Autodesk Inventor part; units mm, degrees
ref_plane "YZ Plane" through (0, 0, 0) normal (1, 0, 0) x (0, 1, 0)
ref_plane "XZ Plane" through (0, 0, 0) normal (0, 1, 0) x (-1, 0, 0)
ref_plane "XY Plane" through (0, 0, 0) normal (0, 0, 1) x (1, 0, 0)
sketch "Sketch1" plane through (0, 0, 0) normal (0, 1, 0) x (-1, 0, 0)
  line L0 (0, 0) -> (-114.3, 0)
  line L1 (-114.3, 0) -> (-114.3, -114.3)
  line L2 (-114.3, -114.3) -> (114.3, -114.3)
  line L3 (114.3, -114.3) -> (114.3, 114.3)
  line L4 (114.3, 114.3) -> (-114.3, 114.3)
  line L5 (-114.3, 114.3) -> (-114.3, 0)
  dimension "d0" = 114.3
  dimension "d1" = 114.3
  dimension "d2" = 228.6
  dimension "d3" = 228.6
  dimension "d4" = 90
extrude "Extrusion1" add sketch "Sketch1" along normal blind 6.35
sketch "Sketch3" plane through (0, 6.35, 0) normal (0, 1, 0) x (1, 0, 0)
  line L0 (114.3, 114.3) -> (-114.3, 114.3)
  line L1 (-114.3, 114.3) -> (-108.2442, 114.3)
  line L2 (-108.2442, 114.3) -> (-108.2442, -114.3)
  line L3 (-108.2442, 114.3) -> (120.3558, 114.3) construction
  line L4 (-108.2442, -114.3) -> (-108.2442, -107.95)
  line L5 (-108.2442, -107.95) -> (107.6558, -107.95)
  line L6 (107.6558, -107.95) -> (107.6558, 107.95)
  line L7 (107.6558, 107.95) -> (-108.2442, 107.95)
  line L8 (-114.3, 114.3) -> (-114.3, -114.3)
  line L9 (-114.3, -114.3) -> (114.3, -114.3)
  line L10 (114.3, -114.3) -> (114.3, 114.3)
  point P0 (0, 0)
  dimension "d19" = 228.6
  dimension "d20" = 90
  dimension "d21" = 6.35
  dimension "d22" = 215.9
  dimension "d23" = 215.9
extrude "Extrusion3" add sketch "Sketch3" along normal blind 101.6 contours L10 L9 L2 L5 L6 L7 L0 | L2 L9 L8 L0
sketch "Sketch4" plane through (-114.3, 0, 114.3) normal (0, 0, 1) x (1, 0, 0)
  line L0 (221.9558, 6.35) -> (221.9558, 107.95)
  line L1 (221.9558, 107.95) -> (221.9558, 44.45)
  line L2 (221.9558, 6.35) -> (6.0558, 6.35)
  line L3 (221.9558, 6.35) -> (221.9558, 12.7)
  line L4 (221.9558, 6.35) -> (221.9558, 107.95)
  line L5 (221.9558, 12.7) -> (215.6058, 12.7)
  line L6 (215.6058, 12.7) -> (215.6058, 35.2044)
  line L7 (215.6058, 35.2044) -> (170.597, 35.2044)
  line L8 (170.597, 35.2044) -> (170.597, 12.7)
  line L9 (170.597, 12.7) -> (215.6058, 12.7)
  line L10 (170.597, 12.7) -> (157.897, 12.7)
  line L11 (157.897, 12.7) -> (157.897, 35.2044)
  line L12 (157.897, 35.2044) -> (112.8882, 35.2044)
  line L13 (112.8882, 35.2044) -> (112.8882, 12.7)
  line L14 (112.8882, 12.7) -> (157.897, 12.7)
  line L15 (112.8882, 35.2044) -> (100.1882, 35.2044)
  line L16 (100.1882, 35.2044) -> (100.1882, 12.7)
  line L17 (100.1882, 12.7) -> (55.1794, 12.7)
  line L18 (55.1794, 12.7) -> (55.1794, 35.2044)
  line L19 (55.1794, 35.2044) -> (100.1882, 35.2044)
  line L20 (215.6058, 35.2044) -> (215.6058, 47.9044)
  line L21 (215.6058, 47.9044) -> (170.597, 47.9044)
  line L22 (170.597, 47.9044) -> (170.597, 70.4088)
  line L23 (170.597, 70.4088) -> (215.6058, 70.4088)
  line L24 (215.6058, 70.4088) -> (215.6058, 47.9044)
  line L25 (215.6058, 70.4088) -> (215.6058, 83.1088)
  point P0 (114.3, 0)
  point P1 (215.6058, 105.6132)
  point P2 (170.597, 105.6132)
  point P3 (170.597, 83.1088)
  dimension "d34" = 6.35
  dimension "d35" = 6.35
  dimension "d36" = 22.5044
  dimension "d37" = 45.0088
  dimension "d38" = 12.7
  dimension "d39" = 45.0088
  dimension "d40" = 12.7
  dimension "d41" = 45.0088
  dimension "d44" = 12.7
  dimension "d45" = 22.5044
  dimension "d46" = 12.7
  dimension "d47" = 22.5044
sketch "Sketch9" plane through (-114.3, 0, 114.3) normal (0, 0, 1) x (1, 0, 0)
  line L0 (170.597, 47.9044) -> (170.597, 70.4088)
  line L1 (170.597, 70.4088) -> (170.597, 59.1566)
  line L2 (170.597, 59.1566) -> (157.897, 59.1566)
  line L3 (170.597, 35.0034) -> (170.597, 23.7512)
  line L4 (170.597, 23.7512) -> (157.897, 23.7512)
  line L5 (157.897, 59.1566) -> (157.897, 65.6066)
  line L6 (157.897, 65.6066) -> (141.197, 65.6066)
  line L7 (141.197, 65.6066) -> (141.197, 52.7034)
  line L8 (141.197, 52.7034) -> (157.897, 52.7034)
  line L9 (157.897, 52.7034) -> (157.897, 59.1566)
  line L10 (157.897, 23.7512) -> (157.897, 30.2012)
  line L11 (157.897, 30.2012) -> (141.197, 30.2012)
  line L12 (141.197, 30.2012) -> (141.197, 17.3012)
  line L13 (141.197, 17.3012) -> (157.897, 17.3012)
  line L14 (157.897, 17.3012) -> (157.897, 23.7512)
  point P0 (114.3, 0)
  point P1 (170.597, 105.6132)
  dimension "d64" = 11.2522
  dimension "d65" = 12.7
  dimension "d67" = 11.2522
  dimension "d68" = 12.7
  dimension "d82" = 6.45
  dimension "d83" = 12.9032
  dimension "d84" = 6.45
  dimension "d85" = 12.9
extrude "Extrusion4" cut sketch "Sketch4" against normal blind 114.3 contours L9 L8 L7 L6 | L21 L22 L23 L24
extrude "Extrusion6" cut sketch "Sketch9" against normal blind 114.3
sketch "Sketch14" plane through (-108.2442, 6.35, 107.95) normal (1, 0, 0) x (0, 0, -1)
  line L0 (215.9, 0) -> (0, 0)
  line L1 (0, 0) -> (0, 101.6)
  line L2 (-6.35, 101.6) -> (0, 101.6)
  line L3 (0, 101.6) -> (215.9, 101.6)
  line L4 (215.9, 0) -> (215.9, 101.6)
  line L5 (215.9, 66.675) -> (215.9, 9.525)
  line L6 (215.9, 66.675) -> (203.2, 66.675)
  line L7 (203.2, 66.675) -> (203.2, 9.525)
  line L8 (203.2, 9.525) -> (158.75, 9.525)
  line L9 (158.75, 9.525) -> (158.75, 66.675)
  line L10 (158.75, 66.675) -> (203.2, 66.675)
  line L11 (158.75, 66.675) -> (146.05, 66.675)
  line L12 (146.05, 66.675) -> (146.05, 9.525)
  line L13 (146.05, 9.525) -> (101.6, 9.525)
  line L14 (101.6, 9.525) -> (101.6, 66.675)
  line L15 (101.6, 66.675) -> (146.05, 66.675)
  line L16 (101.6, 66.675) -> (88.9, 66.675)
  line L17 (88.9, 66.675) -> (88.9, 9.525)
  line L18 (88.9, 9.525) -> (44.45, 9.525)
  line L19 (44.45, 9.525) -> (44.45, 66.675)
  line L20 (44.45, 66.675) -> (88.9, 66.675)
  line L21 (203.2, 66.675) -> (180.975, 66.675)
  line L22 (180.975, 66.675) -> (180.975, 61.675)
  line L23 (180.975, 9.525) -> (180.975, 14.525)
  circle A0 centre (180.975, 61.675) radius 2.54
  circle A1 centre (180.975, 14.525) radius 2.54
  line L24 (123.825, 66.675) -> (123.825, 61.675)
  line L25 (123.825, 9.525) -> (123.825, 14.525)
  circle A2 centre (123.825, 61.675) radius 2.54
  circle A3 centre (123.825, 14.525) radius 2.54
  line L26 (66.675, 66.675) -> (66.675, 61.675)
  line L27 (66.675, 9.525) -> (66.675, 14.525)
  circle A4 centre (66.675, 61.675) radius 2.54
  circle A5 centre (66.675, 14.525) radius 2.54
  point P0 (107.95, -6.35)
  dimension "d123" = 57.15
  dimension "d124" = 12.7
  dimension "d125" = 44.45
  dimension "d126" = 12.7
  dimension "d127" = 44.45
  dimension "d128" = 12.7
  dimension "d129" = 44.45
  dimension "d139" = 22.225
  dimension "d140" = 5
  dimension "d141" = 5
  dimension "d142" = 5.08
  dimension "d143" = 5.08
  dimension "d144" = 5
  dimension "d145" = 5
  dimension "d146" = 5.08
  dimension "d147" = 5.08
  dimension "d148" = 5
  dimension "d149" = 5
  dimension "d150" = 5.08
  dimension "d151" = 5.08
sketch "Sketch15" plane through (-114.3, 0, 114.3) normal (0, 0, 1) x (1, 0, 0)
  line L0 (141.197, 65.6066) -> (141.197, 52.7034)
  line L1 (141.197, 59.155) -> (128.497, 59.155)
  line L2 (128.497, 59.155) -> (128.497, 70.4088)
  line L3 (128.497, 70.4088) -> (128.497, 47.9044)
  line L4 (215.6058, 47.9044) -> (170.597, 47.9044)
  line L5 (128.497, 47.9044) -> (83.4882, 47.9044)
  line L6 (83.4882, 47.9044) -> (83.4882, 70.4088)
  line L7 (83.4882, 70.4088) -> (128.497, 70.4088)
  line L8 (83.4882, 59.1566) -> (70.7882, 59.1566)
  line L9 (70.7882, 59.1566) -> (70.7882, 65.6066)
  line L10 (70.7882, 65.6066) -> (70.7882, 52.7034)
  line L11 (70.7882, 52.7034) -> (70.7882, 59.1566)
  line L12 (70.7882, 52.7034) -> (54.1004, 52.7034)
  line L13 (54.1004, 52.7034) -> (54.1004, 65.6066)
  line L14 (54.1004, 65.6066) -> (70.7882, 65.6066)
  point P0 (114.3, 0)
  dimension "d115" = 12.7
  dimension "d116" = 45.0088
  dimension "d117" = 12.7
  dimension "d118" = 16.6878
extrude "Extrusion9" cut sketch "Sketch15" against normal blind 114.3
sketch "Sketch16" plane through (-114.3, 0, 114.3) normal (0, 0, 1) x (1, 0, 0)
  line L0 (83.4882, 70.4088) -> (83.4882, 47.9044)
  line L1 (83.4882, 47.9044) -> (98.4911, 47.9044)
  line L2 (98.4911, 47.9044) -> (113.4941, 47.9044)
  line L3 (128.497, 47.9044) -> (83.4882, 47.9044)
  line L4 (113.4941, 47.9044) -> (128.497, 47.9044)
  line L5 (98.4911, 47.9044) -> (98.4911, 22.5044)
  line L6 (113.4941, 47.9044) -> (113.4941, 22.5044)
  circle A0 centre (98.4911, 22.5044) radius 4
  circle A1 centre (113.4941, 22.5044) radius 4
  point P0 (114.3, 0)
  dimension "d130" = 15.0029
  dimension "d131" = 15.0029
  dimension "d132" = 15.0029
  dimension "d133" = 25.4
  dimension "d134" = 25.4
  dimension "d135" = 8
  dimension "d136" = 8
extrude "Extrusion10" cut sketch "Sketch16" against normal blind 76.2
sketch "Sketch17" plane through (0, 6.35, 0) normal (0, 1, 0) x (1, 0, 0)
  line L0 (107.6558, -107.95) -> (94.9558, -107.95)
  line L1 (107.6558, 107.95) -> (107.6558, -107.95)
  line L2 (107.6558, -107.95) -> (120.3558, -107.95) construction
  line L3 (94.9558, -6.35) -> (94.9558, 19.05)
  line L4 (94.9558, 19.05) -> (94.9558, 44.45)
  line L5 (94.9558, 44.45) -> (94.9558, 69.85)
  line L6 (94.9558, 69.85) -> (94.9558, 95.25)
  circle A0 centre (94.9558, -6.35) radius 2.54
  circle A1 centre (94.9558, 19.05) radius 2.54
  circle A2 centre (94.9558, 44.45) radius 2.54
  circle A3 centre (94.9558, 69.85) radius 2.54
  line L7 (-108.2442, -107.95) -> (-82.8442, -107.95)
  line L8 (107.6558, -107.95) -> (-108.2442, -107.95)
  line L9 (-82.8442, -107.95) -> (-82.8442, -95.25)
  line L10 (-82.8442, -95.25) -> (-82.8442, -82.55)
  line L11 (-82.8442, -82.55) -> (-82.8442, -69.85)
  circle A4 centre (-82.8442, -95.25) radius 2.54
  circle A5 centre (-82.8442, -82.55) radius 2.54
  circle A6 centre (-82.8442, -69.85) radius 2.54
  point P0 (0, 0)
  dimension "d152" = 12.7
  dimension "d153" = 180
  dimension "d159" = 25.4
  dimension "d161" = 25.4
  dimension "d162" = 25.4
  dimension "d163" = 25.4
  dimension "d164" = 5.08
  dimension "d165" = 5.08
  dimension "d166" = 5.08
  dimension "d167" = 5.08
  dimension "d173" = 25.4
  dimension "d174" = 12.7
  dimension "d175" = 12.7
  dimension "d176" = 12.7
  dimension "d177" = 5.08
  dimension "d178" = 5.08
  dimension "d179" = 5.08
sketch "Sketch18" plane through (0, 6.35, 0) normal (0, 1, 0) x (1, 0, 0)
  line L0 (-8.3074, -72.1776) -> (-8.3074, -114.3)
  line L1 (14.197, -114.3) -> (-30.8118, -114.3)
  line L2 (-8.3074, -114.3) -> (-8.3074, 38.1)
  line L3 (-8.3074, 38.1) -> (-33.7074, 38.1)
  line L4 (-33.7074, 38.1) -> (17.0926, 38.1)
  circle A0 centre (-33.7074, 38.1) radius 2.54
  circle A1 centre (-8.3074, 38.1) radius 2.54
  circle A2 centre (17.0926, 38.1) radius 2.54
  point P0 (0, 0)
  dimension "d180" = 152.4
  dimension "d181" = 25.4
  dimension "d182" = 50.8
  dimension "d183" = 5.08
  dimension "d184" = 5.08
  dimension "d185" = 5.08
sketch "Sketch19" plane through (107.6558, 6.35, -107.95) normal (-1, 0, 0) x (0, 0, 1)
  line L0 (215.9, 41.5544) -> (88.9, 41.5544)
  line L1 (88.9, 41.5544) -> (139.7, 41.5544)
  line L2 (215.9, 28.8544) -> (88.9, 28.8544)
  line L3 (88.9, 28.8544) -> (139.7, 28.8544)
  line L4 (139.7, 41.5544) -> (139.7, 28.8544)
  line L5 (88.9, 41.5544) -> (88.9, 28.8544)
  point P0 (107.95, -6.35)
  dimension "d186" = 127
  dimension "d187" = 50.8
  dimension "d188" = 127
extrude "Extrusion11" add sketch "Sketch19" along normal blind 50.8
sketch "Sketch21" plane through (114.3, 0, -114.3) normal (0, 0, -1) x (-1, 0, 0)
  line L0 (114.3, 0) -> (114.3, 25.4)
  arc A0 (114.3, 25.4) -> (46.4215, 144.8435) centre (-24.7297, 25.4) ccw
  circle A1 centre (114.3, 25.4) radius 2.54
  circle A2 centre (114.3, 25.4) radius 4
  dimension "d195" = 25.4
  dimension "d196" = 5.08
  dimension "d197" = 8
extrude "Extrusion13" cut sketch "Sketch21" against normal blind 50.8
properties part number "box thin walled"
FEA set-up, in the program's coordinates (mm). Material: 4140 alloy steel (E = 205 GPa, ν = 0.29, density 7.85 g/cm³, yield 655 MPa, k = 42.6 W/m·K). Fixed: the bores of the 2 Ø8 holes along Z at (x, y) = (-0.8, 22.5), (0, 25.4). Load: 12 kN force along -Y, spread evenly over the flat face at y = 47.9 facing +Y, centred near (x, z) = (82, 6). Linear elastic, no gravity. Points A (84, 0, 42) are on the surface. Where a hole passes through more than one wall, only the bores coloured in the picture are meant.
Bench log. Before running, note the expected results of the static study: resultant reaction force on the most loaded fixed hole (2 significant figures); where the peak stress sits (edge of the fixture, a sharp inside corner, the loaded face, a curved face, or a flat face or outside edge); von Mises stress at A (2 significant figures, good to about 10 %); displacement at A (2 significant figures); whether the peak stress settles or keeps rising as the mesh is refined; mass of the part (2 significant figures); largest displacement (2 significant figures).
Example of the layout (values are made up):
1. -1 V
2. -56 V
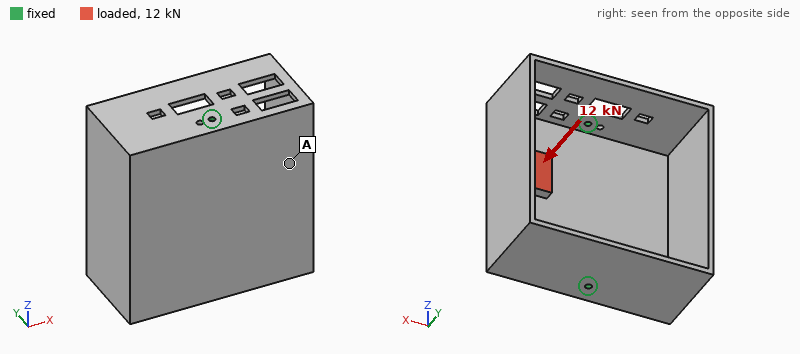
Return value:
1. 6.3 kN
2. edge of the fixture
3. 41 MPa
4. 0.55 mm
5. keeps rising
6. 7.2 kg
7. 1.1 mm
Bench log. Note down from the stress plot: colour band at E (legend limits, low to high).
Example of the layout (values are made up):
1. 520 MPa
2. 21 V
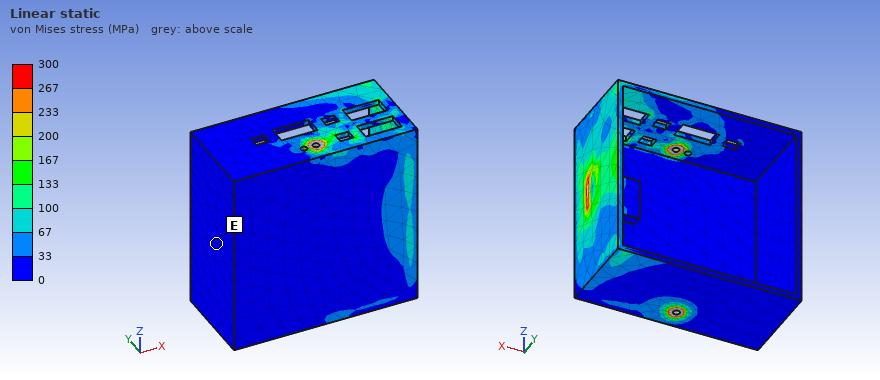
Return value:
1. 0 to 33 MPa
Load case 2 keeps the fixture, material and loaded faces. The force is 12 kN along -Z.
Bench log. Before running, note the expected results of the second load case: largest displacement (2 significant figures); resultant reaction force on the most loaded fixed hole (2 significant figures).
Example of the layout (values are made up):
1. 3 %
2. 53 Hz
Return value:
1. 0.58 mm
2. 7.9 kN
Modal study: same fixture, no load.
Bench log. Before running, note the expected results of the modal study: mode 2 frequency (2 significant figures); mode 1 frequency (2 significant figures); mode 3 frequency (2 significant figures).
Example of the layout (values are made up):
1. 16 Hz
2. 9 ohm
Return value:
1. 400 Hz
2. 290 Hz
3. 670 Hz
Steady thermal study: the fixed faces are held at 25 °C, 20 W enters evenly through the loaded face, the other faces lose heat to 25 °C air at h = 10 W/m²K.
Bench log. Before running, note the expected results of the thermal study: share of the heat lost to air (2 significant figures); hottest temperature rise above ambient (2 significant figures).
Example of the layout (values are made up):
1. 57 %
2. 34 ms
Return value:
1. 83 %
2. 45 K
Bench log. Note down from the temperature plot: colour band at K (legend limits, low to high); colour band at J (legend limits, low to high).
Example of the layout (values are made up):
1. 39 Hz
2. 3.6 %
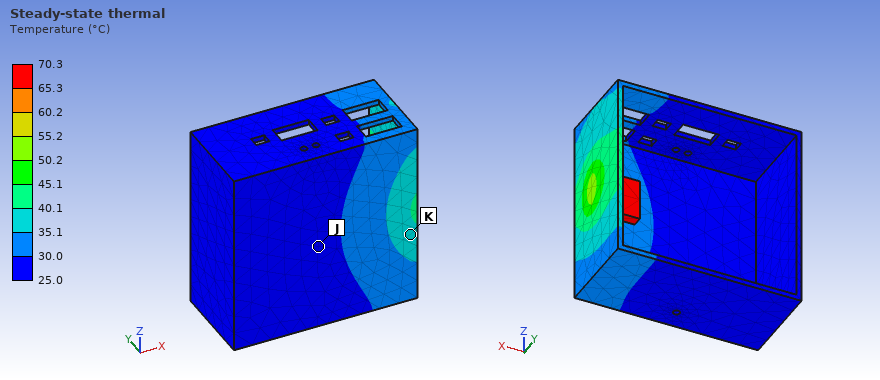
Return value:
1. 35.1 to 40.1 °C
2. 25.0 to 30.0 °C
